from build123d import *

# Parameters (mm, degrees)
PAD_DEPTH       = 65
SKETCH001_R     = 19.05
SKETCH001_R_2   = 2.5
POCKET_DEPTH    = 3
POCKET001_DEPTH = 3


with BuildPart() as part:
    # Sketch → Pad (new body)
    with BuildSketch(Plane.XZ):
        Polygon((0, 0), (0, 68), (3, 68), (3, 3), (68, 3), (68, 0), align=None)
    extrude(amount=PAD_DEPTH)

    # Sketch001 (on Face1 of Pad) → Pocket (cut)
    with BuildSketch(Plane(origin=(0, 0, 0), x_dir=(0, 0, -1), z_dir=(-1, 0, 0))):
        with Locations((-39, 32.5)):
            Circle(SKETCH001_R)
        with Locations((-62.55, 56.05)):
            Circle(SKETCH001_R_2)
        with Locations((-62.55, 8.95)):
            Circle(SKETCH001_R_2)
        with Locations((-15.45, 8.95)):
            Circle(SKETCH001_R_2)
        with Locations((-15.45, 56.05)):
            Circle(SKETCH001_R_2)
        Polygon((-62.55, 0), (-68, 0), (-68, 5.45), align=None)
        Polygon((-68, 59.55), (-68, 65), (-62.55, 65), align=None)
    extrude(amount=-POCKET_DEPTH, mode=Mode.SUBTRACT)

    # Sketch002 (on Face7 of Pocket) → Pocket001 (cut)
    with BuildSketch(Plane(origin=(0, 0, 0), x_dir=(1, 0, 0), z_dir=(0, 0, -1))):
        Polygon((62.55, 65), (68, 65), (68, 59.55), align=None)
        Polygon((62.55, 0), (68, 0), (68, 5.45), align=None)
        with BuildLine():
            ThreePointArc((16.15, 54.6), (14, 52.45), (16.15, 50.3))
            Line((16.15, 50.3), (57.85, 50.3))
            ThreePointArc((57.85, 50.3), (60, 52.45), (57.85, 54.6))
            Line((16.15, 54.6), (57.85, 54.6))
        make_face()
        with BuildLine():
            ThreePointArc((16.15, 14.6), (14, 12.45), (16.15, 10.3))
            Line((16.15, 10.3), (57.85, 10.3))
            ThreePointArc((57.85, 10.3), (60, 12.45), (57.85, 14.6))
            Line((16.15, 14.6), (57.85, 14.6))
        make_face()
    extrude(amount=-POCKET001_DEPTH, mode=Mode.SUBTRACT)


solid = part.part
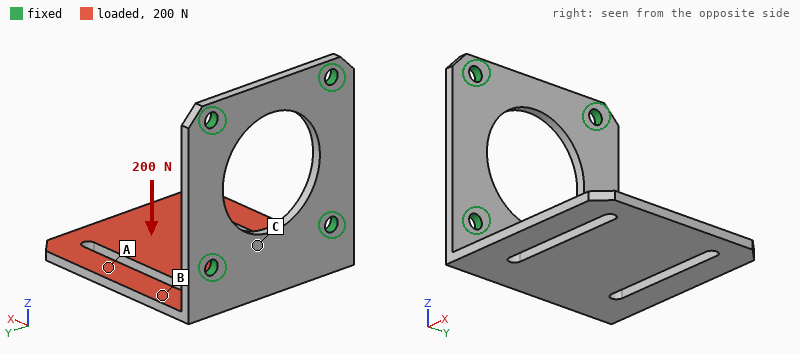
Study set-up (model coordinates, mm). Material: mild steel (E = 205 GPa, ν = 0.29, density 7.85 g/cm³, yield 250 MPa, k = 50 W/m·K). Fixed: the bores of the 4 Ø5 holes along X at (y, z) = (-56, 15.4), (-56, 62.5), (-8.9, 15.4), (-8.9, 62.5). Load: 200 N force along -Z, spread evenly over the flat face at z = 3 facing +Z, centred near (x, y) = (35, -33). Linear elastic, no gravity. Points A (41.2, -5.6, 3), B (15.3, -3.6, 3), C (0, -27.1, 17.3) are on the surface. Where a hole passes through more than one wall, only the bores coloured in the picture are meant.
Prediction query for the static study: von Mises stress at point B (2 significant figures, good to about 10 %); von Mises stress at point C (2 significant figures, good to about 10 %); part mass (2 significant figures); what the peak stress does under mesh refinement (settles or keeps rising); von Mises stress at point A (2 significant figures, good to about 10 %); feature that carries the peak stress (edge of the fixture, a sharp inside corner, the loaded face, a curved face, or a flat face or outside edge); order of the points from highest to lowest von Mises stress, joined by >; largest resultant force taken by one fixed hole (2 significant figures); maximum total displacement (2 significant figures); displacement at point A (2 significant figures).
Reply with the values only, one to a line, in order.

46 MPa
28 MPa
160 g
keeps rising
13 MPa
edge of the fixture
B > C > A
110 N
0.46 mm
0.24 mm
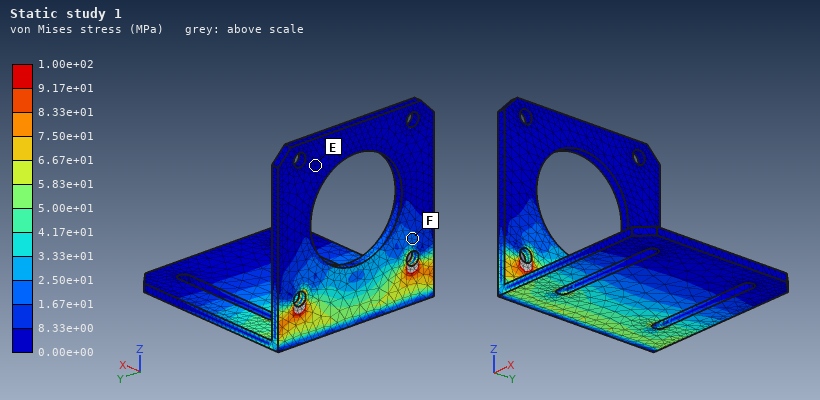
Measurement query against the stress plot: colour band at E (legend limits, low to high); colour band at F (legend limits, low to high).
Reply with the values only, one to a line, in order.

0.00e+00 to 8.33e+00 MPa
1.67e+01 to 2.50e+01 MPa
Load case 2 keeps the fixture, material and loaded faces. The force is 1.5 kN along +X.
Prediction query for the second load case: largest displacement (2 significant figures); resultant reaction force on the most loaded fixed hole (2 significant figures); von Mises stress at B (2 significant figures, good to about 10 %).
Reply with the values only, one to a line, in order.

0.17 mm
770 N
34 MPa
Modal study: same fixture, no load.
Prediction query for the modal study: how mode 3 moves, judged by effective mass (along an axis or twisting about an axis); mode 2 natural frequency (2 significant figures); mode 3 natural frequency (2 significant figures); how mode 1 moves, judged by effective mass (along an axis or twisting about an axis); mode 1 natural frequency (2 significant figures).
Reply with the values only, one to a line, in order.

along Y
1200 Hz
2000 Hz
along Z
430 Hz
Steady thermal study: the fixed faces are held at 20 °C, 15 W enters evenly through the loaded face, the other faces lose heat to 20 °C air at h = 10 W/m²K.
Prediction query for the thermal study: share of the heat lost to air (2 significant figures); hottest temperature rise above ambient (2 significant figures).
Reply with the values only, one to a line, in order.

21 %
68 K
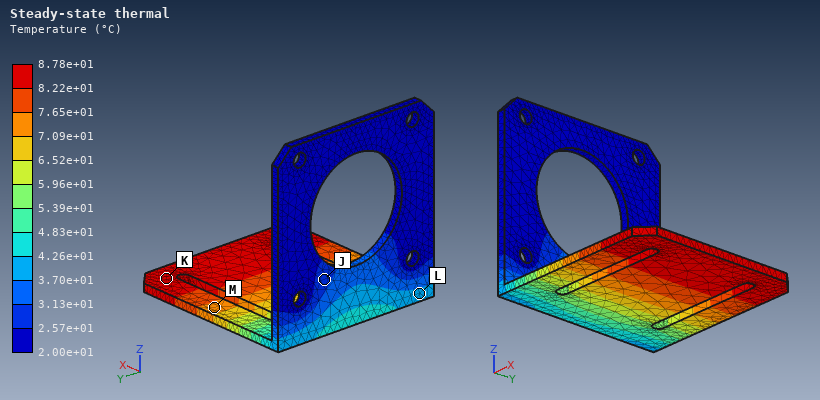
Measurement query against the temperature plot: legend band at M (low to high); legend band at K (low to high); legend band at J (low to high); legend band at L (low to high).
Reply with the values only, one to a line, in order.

7.09e+01 to 7.65e+01 °C
8.22e+01 to 8.78e+01 °C
2.57e+01 to 3.13e+01 °C
3.70e+01 to 4.26e+01 °C
